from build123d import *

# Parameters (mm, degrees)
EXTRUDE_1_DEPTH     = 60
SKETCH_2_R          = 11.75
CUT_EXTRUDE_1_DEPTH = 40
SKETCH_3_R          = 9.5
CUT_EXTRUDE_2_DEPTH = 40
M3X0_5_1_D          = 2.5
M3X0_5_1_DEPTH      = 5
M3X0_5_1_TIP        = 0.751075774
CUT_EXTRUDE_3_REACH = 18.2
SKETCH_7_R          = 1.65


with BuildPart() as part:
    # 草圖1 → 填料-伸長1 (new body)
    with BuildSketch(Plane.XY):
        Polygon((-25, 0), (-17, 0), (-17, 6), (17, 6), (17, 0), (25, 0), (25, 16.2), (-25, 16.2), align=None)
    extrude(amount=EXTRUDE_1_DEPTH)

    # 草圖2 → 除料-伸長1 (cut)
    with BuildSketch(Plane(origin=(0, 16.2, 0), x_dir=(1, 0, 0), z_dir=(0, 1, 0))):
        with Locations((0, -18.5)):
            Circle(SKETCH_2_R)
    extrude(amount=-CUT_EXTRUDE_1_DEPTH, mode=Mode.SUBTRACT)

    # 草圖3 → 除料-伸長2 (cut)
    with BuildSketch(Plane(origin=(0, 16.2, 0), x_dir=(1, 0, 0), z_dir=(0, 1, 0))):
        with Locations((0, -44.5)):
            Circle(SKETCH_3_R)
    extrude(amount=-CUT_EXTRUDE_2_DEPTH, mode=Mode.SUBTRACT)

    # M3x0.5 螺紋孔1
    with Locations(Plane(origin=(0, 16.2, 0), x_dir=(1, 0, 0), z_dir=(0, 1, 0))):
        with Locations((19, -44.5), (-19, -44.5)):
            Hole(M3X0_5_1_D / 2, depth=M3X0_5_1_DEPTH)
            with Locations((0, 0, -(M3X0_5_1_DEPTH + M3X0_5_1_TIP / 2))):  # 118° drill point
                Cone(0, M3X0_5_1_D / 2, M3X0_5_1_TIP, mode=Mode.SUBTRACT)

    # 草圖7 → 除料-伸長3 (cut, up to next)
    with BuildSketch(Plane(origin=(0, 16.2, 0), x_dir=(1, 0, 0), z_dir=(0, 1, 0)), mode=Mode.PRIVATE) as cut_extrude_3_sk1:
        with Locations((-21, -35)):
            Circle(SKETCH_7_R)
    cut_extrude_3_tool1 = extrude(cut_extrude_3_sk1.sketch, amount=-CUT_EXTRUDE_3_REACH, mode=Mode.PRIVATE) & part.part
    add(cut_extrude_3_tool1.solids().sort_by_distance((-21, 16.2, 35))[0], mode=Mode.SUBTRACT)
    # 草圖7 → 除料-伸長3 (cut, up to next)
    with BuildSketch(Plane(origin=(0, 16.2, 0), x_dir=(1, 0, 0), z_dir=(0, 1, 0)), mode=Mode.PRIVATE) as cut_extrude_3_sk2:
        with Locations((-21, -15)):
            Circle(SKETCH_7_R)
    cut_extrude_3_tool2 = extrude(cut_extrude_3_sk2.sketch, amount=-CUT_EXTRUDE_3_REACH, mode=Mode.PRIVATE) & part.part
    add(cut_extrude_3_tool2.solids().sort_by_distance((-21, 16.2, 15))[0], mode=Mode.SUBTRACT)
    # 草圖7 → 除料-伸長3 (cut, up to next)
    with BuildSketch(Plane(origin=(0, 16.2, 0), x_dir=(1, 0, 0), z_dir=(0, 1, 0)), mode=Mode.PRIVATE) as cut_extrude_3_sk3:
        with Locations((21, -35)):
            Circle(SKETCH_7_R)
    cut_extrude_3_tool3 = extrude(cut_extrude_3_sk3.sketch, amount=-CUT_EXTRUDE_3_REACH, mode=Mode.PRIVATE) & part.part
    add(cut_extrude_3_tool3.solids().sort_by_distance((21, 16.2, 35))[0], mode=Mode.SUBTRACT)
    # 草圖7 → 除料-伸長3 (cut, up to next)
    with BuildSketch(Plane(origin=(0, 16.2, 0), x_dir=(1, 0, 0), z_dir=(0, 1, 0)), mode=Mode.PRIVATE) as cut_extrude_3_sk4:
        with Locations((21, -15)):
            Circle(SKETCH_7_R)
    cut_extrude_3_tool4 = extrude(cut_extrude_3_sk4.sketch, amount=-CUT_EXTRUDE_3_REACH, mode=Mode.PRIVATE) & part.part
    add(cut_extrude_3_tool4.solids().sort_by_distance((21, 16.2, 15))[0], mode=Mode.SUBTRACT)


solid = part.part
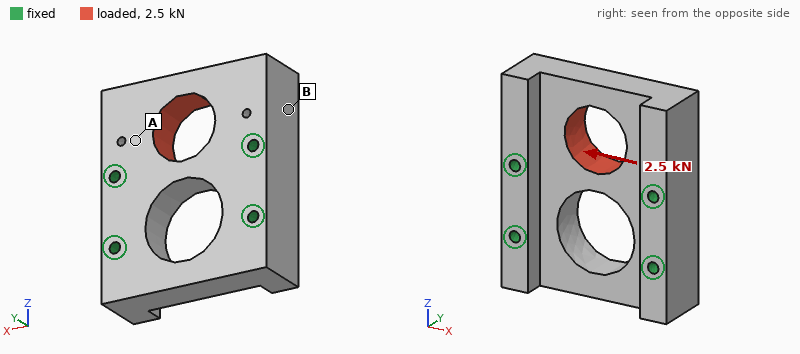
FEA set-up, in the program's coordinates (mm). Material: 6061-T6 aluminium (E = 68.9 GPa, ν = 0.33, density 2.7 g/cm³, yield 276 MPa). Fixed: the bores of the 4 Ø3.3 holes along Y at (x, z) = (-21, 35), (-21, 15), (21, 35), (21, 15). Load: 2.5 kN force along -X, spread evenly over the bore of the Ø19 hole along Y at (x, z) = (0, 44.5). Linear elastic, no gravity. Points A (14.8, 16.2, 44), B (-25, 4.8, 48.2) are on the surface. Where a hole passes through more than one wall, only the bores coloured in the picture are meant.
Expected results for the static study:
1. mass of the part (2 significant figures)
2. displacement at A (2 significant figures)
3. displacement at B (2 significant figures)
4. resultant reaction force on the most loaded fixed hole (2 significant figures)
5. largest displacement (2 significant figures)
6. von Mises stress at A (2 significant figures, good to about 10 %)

77 g
3.6 µm
4.6 µm
1.4 kN
8.2 µm
11 MPa
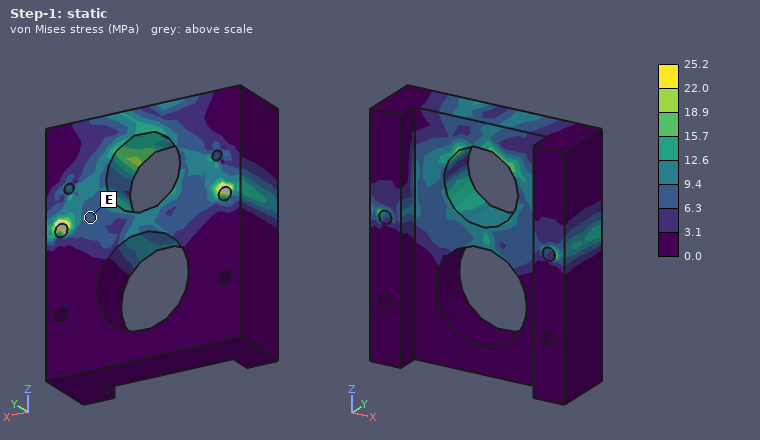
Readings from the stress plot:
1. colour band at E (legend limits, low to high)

6.3 to 9.4 MPa
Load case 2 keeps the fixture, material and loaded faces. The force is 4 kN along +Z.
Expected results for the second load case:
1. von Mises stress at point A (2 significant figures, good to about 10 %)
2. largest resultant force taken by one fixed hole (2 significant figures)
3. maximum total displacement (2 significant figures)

15 MPa
1.4 kN
8.5 µm
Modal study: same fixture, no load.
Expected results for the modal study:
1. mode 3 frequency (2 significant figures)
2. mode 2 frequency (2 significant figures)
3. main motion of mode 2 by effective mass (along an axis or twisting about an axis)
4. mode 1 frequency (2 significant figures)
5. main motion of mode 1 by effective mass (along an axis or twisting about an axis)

18 kHz
15 kHz
along X
12 kHz
along Y
